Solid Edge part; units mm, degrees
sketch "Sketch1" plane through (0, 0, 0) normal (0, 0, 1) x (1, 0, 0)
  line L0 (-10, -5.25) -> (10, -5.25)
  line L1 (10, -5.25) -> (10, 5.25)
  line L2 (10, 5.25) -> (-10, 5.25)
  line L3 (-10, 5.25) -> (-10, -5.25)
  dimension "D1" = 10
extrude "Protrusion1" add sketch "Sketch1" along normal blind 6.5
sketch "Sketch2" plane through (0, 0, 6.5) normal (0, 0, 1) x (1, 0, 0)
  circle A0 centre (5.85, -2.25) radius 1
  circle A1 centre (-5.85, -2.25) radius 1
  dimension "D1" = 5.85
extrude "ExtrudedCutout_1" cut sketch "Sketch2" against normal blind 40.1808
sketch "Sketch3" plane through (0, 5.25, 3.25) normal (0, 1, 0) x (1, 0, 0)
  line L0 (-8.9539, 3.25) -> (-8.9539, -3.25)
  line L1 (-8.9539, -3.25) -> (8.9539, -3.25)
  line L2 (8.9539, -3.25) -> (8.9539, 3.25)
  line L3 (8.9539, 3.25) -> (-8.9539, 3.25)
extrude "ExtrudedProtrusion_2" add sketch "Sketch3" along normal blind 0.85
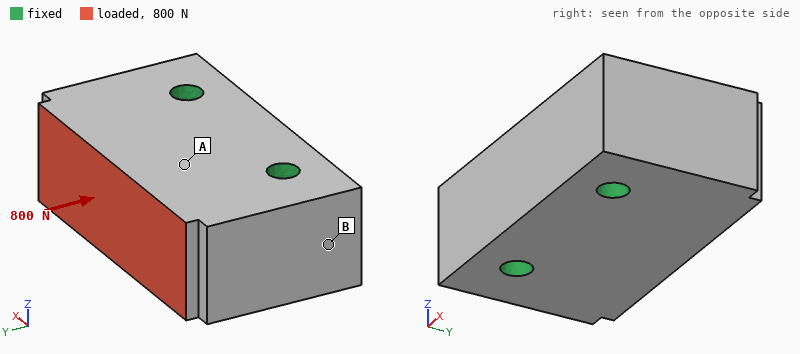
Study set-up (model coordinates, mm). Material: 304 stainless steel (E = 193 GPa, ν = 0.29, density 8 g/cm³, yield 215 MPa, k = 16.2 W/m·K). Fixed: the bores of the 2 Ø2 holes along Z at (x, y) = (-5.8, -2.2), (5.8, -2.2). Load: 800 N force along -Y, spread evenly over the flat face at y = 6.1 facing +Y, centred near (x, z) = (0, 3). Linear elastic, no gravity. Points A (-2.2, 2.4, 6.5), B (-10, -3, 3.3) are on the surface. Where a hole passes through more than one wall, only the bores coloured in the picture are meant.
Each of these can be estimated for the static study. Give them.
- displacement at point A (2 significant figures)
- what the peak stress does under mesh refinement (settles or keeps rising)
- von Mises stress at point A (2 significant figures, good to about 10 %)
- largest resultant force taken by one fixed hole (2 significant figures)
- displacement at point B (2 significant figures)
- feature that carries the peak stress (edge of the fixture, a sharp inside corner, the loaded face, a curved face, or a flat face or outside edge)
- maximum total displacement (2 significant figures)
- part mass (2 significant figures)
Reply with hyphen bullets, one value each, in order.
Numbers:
- 0.27 µm
- keeps rising
- 6.1 MPa
- 410 N
- 0.12 µm
- edge of the fixture
- 0.40 µm
- 11 g
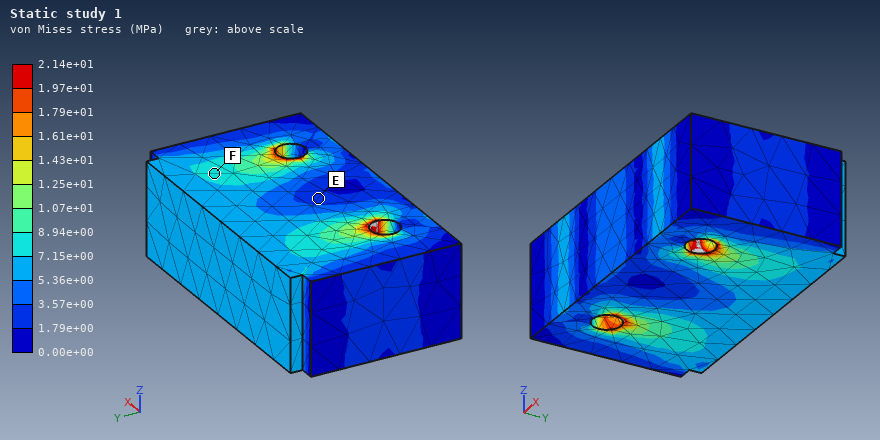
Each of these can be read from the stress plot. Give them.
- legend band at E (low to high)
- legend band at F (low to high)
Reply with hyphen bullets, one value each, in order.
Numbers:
- 1.79e+00 to 3.57e+00 MPa
- 7.15e+00 to 8.94e+00 MPa
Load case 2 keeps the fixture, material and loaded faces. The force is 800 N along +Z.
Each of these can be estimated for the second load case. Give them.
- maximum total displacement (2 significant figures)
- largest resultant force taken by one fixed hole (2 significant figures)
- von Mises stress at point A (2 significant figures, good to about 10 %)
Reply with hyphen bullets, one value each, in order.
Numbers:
- 4.0 µm
- 400 N
- 20 MPa
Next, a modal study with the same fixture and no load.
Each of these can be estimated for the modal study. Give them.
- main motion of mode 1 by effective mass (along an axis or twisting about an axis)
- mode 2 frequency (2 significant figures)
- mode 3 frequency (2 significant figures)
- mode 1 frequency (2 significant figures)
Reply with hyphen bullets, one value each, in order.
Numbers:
- along Z
- 65 kHz
- 67 kHz
- 46 kHz
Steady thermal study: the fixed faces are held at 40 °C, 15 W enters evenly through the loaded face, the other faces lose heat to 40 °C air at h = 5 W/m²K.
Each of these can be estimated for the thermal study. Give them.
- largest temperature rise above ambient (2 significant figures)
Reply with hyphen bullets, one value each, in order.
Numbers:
- 69 K
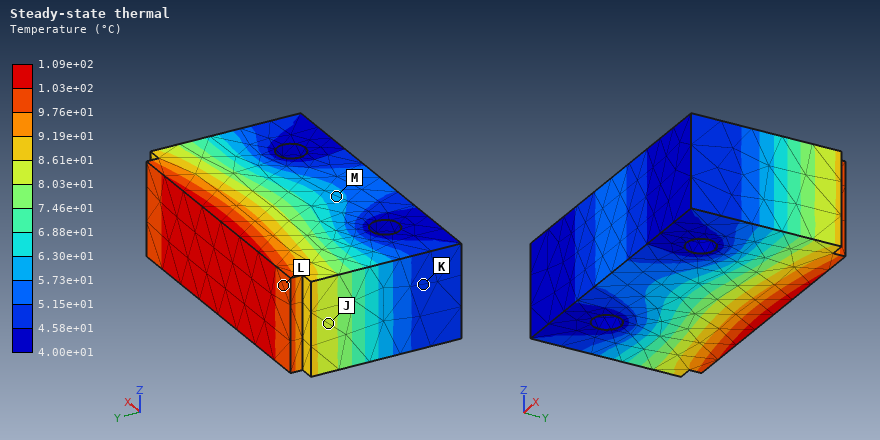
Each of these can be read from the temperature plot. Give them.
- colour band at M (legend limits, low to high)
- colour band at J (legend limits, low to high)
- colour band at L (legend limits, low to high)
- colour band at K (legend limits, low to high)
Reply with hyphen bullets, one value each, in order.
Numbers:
- 5.73e+01 to 6.30e+01 °C
- 8.03e+01 to 8.61e+01 °C
- 9.76e+01 to 1.03e+02 °C
- 4.58e+01 to 5.15e+01 °C
